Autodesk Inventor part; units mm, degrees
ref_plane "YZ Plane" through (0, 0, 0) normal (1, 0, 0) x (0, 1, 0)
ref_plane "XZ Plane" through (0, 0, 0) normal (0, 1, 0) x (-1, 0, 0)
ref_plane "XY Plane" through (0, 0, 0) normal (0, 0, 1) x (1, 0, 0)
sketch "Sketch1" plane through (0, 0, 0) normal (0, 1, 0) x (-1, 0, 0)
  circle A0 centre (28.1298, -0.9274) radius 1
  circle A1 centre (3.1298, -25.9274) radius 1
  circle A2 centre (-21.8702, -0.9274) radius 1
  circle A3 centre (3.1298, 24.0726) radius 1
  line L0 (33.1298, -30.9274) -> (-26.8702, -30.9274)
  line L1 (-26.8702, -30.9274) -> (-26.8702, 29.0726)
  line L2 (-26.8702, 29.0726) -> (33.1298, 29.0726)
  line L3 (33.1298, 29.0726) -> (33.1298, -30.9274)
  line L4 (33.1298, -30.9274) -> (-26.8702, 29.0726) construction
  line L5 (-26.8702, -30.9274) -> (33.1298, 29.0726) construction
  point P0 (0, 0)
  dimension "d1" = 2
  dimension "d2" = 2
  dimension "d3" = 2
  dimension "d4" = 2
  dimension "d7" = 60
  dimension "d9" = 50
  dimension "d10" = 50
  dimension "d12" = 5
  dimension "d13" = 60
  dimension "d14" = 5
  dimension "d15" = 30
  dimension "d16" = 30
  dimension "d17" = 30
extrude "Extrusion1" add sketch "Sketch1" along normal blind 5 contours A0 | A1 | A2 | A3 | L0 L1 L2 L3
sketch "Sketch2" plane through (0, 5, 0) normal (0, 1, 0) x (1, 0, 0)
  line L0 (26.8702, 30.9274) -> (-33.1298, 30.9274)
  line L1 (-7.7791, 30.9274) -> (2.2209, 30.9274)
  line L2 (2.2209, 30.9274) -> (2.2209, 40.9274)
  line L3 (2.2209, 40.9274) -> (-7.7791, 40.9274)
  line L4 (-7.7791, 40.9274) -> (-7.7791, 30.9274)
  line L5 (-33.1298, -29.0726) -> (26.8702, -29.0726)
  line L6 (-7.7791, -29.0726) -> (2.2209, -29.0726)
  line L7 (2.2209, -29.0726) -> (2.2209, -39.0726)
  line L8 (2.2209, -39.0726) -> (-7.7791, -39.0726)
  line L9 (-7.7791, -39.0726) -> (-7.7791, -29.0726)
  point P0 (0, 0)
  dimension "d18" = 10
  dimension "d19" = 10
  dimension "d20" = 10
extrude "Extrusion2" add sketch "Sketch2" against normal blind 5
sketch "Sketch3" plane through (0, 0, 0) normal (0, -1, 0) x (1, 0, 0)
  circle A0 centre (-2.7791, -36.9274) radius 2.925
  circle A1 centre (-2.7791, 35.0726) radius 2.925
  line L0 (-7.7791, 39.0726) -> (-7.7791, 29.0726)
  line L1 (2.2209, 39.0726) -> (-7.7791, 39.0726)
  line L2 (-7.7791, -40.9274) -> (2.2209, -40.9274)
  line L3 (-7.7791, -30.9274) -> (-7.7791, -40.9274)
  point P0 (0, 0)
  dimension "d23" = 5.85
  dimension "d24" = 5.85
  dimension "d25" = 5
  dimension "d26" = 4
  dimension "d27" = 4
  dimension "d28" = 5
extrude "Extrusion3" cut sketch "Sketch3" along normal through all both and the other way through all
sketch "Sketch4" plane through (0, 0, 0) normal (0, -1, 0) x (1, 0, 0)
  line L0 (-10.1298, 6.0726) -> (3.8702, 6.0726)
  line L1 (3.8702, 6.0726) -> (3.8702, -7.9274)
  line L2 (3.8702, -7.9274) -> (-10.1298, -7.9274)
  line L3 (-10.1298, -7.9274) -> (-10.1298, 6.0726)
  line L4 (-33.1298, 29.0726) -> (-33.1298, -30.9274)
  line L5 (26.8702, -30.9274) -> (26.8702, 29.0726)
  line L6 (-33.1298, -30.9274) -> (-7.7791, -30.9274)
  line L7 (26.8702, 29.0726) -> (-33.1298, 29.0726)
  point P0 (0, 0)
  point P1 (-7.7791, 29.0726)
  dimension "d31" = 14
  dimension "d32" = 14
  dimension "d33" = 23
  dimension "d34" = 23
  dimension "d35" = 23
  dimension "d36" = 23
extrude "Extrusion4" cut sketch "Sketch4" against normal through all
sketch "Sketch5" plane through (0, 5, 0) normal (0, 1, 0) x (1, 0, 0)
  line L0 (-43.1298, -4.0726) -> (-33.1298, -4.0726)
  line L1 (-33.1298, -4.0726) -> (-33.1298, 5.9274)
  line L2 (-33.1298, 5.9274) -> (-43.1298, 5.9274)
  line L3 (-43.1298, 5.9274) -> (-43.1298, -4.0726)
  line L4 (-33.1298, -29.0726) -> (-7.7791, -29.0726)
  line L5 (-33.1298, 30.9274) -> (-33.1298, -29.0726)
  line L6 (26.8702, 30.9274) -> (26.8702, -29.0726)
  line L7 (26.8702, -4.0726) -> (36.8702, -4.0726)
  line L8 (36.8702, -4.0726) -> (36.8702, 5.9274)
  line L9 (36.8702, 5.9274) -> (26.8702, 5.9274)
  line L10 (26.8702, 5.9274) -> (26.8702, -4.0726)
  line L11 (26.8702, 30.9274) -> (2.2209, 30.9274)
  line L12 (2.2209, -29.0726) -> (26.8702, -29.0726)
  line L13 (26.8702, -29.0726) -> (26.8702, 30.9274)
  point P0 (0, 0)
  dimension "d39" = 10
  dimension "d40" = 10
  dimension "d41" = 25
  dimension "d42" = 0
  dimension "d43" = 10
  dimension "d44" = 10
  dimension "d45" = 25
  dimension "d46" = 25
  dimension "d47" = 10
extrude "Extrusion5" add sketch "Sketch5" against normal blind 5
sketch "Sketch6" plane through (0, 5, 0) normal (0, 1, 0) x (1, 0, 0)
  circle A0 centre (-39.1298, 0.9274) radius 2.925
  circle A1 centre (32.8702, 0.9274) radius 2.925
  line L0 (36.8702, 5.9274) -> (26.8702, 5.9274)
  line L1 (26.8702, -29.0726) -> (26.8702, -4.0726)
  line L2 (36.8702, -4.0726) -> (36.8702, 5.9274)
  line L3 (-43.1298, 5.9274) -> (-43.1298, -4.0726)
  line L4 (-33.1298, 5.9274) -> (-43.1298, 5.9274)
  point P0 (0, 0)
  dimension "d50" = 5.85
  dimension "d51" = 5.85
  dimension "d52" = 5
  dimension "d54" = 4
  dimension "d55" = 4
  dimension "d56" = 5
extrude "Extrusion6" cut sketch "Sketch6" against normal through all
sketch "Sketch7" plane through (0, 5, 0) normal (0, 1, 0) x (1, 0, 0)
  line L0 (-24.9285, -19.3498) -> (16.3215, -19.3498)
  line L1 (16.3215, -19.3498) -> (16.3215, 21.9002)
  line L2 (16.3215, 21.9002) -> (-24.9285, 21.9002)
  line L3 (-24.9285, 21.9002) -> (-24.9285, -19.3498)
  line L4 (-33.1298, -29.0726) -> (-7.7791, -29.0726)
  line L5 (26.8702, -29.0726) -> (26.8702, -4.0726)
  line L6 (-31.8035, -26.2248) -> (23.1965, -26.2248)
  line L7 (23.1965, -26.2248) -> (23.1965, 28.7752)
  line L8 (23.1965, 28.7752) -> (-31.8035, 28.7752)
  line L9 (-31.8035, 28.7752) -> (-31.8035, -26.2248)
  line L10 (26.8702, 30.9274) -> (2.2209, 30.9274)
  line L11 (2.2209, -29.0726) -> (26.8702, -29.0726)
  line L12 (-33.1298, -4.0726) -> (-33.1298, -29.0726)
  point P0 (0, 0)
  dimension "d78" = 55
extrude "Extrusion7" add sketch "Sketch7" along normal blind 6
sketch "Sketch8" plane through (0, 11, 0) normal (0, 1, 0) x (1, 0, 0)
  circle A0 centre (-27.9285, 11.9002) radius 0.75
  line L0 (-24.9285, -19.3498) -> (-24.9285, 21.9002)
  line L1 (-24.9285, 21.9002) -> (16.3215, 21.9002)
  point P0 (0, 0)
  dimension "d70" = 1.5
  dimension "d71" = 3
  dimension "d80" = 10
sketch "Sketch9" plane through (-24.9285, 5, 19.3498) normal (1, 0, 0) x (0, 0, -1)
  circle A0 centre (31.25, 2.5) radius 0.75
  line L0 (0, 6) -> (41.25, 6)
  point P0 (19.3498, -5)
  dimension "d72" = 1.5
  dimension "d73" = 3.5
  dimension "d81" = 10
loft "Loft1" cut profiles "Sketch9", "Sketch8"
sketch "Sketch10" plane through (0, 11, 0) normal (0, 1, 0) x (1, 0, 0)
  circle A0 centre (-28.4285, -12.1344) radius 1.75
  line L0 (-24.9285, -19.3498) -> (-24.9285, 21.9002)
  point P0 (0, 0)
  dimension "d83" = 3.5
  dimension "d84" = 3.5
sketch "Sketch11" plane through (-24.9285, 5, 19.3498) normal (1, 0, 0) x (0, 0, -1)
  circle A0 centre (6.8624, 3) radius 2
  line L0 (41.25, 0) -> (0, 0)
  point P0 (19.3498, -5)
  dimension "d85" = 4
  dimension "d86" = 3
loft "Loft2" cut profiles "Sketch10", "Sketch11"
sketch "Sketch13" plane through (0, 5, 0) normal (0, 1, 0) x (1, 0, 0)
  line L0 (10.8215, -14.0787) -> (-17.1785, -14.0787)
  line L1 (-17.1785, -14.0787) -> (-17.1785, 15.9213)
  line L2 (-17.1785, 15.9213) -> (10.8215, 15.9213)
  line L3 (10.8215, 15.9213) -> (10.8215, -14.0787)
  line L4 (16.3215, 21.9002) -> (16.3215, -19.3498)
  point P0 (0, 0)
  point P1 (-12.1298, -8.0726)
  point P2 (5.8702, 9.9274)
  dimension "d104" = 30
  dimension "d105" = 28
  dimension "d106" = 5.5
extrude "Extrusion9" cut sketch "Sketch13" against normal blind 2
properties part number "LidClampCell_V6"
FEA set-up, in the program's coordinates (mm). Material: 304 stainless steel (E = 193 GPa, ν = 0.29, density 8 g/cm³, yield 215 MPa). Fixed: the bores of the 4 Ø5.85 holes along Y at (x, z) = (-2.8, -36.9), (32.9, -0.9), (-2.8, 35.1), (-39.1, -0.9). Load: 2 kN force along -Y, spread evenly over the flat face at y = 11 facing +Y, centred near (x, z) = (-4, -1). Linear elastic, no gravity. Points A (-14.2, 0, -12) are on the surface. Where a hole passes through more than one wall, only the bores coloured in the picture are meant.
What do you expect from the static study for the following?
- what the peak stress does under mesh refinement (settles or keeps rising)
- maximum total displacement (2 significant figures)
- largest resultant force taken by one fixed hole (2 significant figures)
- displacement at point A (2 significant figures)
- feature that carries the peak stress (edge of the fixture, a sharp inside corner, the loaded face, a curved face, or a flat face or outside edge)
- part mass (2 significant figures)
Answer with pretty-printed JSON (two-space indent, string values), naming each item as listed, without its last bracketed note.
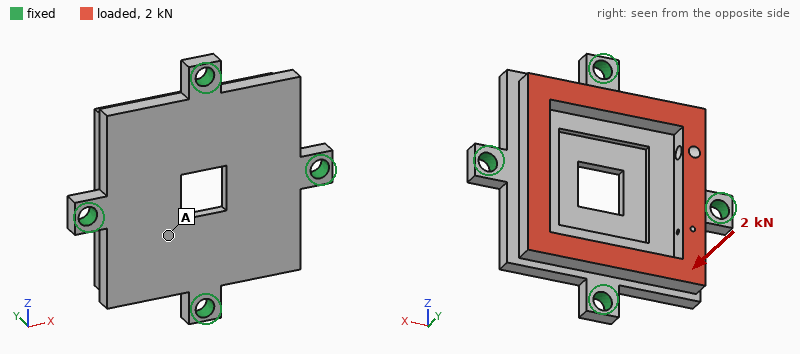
{
  "what the peak stress does under mesh refinement": "keeps rising",
  "maximum total displacement": "5.6 µm",
  "largest resultant force taken by one fixed hole": "530 N",
  "displacement at point A": "4.6 µm",
  "feature that carries the peak stress": "edge of the fixture",
  "part mass": "200 g"
}
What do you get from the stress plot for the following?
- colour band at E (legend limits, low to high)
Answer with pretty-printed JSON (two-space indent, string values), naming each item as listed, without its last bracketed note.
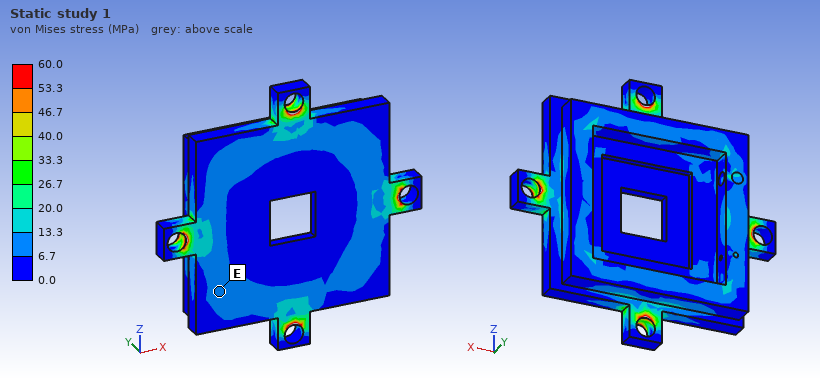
{
  "colour band at E": "6.7 to 13.3 MPa"
}
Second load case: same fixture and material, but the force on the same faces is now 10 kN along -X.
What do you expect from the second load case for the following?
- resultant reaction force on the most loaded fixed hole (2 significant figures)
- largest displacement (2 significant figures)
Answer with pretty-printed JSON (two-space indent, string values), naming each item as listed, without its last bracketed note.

{
  "resultant reaction force on the most loaded fixed hole": "3.3 kN",
  "largest displacement": "21 µm"
}
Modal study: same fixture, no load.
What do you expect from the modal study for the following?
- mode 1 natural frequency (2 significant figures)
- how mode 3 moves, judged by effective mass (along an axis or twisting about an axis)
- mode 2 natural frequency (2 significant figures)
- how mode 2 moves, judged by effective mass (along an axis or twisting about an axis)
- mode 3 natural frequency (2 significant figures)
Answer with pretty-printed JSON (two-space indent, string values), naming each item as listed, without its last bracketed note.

{
  "mode 1 natural frequency": "6100 Hz",
  "how mode 3 moves, judged by effective mass": "twisting about Z",
  "mode 2 natural frequency": "7600 Hz",
  "how mode 2 moves, judged by effective mass": "along Y",
  "mode 3 natural frequency": "8300 Hz"
}
